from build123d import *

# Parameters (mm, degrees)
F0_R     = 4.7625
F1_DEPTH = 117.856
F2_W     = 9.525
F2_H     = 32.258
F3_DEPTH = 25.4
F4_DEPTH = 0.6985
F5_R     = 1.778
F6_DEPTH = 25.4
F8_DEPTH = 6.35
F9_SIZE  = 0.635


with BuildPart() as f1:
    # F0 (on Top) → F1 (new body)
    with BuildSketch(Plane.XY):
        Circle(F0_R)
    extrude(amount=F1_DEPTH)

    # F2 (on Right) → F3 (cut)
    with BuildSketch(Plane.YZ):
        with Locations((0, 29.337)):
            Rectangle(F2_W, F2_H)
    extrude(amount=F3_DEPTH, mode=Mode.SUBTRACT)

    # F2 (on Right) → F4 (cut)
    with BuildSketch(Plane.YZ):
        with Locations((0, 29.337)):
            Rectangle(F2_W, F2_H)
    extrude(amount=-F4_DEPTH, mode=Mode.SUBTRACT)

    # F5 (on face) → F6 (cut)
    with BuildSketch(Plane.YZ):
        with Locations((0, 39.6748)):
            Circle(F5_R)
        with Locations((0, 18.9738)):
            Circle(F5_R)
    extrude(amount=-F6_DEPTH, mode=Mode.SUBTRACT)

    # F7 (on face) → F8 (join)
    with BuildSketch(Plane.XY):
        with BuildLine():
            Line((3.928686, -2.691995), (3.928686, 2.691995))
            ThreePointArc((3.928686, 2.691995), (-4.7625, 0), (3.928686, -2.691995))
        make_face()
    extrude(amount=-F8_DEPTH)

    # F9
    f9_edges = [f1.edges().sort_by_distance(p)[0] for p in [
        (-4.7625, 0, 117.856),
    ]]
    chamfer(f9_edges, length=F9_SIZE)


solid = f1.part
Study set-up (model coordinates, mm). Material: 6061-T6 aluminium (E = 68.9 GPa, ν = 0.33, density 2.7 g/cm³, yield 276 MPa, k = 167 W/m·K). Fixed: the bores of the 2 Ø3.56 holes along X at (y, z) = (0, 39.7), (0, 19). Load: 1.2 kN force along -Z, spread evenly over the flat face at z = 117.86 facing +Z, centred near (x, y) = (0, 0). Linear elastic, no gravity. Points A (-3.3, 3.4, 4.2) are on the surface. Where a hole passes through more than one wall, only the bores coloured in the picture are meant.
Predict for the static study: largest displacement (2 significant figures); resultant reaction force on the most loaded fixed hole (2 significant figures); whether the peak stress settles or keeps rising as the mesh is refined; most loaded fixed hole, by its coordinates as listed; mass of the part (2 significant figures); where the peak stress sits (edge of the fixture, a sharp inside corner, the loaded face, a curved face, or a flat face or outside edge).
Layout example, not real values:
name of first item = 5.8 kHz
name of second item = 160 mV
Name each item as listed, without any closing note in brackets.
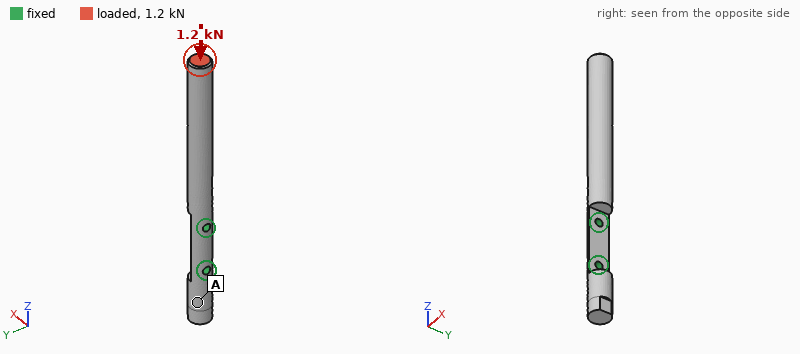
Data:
largest displacement = 0.59 mm
resultant reaction force on the most loaded fixed hole = 1.1 kN
whether the peak stress settles or keeps rising as the mesh is refined = keeps rising
most loaded fixed hole, by its coordinates as listed = (0, 39.7)
mass of the part = 20 g
where the peak stress sits = edge of the fixture
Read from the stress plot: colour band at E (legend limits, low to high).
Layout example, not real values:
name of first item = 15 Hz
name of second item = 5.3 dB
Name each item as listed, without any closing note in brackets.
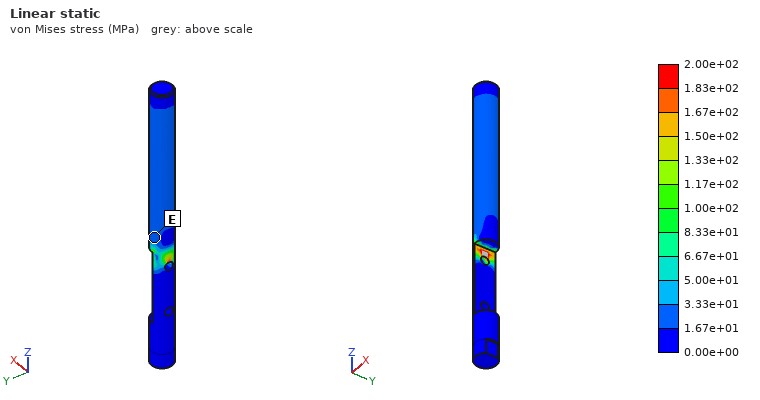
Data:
colour band at E = 1.67e+01 to 3.33e+01 MPa
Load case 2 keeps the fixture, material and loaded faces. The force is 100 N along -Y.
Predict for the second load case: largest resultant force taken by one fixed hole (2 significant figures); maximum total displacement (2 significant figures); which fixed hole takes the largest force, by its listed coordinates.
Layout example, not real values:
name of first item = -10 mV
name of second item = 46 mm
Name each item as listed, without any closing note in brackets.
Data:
largest resultant force taken by one fixed hole = 200 N
maximum total displacement = 0.91 mm
which fixed hole takes the largest force, by its listed coordinates = (0, 39.7)
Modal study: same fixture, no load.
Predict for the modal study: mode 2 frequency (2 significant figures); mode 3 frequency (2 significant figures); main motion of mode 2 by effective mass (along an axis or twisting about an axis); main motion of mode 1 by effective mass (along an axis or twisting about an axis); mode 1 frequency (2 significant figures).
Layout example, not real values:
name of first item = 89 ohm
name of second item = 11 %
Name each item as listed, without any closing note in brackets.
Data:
mode 2 frequency = 830 Hz
mode 3 frequency = 3700 Hz
main motion of mode 2 by effective mass = along Y
main motion of mode 1 by effective mass = along X
mode 1 frequency = 550 Hz
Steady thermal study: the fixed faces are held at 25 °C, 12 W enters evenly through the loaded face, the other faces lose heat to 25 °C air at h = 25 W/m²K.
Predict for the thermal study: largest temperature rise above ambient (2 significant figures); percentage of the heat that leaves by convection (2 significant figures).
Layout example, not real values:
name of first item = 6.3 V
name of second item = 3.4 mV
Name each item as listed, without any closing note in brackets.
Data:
largest temperature rise above ambient = 77 K
percentage of the heat that leaves by convection = 20 %
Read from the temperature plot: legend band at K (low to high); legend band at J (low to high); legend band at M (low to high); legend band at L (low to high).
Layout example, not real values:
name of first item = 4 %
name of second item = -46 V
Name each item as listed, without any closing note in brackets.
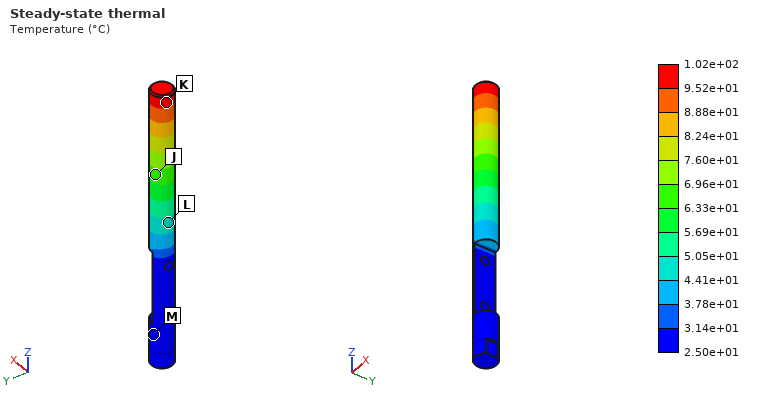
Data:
legend band at K = 9.52e+01 to 1.02e+02 °C
legend band at J = 6.33e+01 to 6.96e+01 °C
legend band at M = 2.50e+01 to 3.14e+01 °C
legend band at L = 4.41e+01 to 5.05e+01 °C
